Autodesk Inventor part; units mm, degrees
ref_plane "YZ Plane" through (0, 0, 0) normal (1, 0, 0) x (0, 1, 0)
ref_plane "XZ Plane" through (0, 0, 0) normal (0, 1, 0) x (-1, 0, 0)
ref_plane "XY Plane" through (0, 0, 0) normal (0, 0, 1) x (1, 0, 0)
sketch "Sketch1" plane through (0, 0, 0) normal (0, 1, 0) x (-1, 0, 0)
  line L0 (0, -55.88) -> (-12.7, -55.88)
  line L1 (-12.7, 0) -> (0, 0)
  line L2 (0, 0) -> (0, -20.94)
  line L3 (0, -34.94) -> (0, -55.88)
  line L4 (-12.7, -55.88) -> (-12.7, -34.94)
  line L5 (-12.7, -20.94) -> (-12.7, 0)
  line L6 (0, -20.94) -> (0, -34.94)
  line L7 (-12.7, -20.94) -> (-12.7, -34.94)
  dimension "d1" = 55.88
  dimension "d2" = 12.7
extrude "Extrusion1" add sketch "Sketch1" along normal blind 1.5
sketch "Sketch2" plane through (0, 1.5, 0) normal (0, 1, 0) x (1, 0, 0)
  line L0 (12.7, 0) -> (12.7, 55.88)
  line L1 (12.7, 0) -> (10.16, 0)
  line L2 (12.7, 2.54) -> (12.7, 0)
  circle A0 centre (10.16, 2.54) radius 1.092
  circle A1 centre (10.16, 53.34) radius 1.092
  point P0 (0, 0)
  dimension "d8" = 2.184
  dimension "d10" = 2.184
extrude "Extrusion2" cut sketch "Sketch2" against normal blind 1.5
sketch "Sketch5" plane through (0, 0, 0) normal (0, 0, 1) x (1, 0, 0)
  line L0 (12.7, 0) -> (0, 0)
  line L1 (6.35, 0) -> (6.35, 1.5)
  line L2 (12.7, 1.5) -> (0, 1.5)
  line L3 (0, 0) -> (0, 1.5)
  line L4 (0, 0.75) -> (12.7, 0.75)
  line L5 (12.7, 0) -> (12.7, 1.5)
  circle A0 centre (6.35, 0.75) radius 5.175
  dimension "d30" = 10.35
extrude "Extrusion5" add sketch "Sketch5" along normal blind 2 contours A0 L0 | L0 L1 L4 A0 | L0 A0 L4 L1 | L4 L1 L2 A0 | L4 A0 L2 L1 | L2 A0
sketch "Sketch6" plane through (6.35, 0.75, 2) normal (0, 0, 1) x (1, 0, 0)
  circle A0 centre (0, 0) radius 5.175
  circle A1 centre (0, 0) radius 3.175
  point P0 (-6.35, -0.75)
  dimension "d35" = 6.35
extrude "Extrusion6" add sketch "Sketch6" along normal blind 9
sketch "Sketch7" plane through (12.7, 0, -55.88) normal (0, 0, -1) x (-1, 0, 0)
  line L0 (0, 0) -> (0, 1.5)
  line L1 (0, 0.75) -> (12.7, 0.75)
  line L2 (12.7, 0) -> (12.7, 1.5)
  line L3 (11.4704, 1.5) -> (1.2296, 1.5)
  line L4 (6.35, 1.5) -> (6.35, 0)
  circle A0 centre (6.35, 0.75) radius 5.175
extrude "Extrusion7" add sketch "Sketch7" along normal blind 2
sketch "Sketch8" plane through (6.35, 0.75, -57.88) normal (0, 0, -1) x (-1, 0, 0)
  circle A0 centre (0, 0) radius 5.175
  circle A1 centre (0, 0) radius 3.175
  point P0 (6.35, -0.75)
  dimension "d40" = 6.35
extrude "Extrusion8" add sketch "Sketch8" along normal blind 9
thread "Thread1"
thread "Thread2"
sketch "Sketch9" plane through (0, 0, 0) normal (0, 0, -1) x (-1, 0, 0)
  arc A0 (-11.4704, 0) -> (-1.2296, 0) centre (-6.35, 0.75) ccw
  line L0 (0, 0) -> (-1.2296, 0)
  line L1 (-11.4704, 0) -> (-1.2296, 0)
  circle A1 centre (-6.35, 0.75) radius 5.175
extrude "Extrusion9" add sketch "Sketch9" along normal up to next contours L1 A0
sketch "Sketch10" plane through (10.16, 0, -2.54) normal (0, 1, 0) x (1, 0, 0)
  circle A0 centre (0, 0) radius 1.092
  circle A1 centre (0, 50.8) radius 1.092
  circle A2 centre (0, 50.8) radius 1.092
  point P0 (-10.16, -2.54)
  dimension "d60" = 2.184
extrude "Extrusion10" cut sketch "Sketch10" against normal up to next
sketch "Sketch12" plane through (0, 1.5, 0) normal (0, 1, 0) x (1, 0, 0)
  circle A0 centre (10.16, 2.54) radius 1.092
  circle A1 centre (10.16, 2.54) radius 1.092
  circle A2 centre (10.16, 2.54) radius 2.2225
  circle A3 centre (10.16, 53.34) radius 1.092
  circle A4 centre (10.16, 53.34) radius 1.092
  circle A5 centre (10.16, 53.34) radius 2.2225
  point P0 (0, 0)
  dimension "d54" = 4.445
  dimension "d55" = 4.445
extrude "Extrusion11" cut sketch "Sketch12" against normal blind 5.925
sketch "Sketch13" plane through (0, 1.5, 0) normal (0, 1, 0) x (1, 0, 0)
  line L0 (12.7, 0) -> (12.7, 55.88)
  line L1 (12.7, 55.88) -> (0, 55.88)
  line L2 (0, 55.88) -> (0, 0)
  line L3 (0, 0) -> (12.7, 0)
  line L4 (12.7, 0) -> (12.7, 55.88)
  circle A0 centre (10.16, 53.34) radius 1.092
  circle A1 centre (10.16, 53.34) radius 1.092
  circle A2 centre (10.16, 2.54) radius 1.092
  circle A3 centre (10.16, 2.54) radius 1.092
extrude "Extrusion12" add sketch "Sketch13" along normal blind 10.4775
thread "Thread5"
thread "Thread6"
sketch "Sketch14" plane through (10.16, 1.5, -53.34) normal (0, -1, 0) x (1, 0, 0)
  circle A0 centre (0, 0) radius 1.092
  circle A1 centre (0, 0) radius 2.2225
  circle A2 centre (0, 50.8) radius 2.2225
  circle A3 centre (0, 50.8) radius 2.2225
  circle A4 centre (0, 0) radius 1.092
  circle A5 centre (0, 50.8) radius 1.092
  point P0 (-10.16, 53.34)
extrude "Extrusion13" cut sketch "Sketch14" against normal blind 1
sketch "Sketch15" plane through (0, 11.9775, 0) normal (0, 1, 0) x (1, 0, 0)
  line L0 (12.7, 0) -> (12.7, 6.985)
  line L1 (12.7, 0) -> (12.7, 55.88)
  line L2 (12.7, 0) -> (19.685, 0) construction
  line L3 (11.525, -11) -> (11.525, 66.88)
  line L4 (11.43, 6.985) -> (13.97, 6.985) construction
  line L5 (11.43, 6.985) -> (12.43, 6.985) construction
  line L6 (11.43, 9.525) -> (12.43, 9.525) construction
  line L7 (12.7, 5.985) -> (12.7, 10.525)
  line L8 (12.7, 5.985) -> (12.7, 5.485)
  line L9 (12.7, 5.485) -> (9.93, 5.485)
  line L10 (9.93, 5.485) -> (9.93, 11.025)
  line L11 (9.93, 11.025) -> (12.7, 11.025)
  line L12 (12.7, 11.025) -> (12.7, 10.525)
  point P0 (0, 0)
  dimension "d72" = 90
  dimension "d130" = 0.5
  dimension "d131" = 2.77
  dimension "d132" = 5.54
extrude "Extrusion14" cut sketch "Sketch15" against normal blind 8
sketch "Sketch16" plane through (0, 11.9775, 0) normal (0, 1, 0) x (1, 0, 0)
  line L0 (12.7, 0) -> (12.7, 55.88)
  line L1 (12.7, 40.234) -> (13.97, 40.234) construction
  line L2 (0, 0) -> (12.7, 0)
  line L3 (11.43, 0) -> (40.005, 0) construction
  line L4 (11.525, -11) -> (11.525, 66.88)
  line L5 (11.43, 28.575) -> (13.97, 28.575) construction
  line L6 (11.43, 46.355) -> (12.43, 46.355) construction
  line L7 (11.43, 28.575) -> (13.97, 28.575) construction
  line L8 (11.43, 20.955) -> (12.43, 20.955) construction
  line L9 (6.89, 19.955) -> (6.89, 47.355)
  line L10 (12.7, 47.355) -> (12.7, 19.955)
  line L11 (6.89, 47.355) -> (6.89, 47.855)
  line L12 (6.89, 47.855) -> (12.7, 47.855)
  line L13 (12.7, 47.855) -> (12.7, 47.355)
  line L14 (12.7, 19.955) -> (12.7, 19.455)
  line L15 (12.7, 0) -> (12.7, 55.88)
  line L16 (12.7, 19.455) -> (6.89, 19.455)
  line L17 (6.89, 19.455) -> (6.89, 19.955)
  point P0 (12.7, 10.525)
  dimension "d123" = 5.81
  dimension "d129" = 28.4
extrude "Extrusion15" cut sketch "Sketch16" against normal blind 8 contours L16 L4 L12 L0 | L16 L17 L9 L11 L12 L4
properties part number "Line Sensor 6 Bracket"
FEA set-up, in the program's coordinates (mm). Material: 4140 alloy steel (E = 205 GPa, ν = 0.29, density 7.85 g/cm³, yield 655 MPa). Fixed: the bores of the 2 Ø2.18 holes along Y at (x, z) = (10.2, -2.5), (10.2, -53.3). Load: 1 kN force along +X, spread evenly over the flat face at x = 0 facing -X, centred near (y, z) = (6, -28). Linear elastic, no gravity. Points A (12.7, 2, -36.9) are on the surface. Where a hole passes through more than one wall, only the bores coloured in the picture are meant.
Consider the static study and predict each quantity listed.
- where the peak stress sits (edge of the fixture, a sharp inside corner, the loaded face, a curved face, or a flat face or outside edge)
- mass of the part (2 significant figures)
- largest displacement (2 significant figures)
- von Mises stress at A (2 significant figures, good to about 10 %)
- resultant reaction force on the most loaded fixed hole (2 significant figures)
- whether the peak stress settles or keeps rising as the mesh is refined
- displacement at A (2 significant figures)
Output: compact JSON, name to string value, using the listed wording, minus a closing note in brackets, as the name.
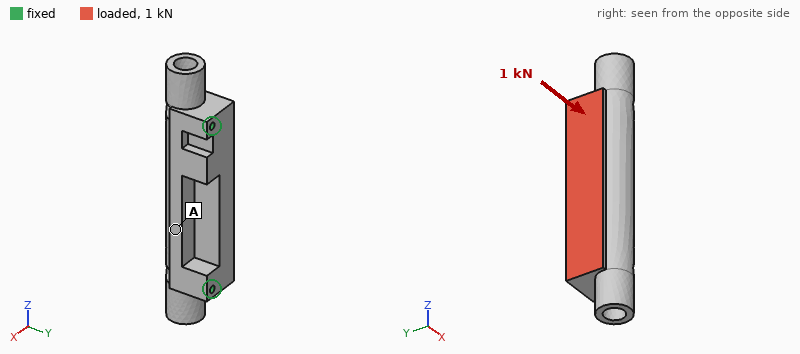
{"where the peak stress sits": "edge of the fixture", "mass of the part": "79 g", "largest displacement": "3.3 µm", "von Mises stress at A": "7.8 MPa", "resultant reaction force on the most loaded fixed hole": "650 N", "whether the peak stress settles or keeps rising as the mesh is refined": "keeps rising", "displacement at A": "2.4 µm"}
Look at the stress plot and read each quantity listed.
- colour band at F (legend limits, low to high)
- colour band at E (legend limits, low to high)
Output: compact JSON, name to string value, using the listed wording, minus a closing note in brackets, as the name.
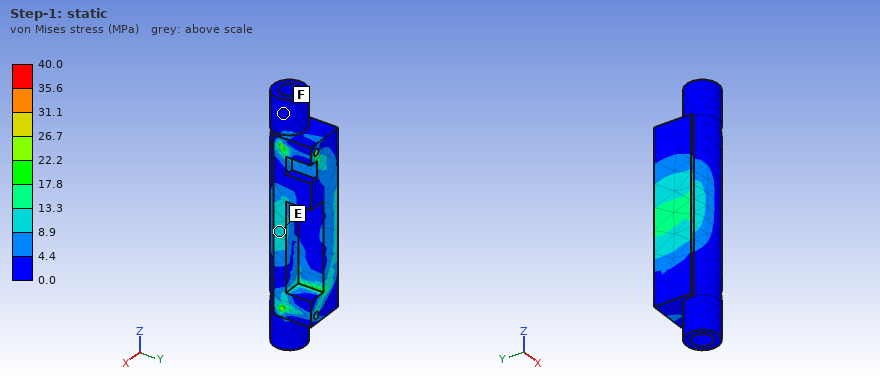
{"colour band at F": "0.0 to 4.4 MPa", "colour band at E": "8.9 to 13.3 MPa"}
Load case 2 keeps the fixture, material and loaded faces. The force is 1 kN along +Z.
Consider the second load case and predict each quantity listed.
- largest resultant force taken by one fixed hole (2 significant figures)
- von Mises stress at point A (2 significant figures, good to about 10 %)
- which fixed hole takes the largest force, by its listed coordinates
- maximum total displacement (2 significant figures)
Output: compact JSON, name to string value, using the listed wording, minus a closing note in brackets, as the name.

{"largest resultant force taken by one fixed hole": "560 N", "von Mises stress at point A": "4.5 MPa", "which fixed hole takes the largest force, by its listed coordinates": "(10.2, -2.5)", "maximum total displacement": "1.5 µm"}
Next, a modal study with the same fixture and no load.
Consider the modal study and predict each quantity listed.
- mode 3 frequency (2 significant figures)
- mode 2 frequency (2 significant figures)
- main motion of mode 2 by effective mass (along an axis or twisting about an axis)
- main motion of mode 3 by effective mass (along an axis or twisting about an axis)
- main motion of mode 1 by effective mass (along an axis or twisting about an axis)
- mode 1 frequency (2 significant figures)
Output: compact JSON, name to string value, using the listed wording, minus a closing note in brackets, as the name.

{"mode 3 frequency": "18 kHz", "mode 2 frequency": "14 kHz", "main motion of mode 2 by effective mass": "along Y", "main motion of mode 3 by effective mass": "twisting about Z", "main motion of mode 1 by effective mass": "along X", "mode 1 frequency": "12 kHz"}
